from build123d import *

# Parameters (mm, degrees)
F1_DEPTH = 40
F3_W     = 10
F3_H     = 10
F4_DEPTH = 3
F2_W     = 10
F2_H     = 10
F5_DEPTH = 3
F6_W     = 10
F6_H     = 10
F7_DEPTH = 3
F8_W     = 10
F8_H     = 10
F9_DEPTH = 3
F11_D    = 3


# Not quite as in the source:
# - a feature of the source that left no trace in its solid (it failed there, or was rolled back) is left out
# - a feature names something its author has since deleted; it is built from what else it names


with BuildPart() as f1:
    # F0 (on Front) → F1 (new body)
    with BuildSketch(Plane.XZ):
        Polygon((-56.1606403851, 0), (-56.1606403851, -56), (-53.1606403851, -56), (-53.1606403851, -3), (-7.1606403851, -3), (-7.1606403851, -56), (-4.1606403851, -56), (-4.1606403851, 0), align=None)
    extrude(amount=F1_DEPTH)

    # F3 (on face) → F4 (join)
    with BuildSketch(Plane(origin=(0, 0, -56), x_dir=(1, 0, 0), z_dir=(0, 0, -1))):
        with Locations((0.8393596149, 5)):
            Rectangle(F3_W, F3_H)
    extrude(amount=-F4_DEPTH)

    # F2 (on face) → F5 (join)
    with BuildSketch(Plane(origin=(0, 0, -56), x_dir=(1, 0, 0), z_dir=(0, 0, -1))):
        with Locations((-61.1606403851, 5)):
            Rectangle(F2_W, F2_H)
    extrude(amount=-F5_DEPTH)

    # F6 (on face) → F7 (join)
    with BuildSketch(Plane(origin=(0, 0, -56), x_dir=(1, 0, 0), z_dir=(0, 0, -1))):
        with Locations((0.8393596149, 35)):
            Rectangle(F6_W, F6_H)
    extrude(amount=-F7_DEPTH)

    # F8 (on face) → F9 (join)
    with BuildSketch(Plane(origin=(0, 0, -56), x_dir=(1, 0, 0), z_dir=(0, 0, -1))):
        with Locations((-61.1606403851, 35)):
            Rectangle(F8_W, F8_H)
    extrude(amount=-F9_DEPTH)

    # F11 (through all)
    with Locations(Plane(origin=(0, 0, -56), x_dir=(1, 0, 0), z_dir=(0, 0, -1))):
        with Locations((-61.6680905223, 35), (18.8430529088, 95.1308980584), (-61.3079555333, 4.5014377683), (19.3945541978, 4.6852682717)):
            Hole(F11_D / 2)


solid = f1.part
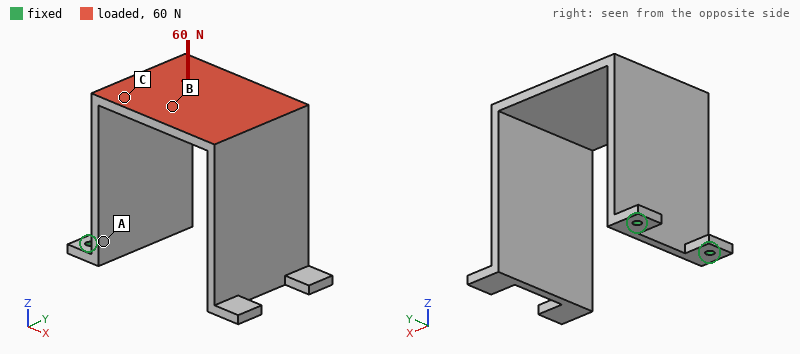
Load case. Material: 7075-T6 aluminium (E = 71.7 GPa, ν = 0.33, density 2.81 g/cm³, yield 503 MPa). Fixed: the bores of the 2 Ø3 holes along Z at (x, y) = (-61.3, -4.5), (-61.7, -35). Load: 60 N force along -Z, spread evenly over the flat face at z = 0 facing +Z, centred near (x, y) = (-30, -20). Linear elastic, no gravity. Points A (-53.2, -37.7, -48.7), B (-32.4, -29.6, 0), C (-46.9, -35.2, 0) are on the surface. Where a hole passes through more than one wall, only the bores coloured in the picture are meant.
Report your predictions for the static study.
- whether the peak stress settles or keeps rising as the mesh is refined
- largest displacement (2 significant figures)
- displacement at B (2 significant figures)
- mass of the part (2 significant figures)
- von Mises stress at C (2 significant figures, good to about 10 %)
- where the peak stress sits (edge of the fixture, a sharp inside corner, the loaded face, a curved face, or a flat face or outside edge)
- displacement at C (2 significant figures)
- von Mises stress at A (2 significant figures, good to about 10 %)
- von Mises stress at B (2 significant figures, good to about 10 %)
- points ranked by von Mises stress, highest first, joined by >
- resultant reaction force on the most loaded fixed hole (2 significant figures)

keeps rising
1.2 mm
0.64 mm
57 g
16 MPa
edge of the fixture
0.53 mm
33 MPa
7.1 MPa
A > C > B
31 N
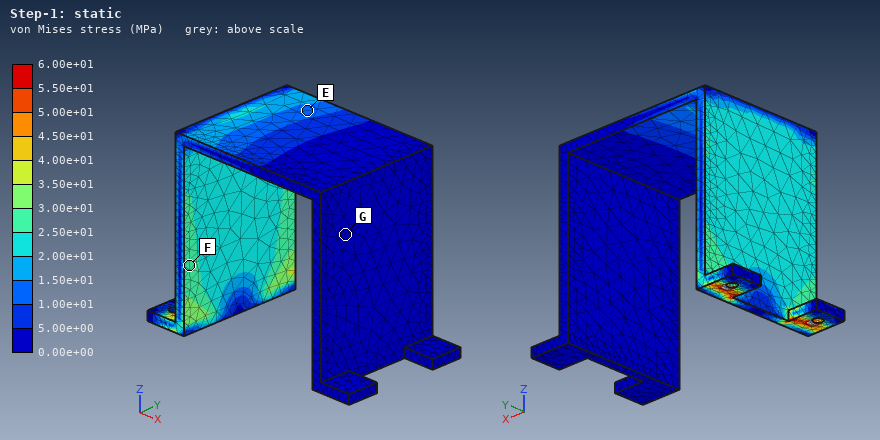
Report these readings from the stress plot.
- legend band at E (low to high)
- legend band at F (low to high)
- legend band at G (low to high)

1.00e+01 to 1.50e+01 MPa
2.50e+01 to 3.00e+01 MPa
0.00e+00 to 5.00e+00 MPa
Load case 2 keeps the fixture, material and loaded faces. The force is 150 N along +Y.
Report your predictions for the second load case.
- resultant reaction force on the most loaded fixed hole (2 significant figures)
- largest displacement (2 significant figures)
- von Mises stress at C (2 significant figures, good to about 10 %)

300 N
1.1 mm
15 MPa
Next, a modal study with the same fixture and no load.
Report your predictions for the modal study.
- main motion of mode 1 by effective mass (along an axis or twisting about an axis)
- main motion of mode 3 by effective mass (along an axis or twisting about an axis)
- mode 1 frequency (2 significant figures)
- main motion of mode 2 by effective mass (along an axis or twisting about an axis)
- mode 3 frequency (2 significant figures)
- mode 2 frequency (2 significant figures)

along Z
along X
150 Hz
along Y
300 Hz
250 Hz
